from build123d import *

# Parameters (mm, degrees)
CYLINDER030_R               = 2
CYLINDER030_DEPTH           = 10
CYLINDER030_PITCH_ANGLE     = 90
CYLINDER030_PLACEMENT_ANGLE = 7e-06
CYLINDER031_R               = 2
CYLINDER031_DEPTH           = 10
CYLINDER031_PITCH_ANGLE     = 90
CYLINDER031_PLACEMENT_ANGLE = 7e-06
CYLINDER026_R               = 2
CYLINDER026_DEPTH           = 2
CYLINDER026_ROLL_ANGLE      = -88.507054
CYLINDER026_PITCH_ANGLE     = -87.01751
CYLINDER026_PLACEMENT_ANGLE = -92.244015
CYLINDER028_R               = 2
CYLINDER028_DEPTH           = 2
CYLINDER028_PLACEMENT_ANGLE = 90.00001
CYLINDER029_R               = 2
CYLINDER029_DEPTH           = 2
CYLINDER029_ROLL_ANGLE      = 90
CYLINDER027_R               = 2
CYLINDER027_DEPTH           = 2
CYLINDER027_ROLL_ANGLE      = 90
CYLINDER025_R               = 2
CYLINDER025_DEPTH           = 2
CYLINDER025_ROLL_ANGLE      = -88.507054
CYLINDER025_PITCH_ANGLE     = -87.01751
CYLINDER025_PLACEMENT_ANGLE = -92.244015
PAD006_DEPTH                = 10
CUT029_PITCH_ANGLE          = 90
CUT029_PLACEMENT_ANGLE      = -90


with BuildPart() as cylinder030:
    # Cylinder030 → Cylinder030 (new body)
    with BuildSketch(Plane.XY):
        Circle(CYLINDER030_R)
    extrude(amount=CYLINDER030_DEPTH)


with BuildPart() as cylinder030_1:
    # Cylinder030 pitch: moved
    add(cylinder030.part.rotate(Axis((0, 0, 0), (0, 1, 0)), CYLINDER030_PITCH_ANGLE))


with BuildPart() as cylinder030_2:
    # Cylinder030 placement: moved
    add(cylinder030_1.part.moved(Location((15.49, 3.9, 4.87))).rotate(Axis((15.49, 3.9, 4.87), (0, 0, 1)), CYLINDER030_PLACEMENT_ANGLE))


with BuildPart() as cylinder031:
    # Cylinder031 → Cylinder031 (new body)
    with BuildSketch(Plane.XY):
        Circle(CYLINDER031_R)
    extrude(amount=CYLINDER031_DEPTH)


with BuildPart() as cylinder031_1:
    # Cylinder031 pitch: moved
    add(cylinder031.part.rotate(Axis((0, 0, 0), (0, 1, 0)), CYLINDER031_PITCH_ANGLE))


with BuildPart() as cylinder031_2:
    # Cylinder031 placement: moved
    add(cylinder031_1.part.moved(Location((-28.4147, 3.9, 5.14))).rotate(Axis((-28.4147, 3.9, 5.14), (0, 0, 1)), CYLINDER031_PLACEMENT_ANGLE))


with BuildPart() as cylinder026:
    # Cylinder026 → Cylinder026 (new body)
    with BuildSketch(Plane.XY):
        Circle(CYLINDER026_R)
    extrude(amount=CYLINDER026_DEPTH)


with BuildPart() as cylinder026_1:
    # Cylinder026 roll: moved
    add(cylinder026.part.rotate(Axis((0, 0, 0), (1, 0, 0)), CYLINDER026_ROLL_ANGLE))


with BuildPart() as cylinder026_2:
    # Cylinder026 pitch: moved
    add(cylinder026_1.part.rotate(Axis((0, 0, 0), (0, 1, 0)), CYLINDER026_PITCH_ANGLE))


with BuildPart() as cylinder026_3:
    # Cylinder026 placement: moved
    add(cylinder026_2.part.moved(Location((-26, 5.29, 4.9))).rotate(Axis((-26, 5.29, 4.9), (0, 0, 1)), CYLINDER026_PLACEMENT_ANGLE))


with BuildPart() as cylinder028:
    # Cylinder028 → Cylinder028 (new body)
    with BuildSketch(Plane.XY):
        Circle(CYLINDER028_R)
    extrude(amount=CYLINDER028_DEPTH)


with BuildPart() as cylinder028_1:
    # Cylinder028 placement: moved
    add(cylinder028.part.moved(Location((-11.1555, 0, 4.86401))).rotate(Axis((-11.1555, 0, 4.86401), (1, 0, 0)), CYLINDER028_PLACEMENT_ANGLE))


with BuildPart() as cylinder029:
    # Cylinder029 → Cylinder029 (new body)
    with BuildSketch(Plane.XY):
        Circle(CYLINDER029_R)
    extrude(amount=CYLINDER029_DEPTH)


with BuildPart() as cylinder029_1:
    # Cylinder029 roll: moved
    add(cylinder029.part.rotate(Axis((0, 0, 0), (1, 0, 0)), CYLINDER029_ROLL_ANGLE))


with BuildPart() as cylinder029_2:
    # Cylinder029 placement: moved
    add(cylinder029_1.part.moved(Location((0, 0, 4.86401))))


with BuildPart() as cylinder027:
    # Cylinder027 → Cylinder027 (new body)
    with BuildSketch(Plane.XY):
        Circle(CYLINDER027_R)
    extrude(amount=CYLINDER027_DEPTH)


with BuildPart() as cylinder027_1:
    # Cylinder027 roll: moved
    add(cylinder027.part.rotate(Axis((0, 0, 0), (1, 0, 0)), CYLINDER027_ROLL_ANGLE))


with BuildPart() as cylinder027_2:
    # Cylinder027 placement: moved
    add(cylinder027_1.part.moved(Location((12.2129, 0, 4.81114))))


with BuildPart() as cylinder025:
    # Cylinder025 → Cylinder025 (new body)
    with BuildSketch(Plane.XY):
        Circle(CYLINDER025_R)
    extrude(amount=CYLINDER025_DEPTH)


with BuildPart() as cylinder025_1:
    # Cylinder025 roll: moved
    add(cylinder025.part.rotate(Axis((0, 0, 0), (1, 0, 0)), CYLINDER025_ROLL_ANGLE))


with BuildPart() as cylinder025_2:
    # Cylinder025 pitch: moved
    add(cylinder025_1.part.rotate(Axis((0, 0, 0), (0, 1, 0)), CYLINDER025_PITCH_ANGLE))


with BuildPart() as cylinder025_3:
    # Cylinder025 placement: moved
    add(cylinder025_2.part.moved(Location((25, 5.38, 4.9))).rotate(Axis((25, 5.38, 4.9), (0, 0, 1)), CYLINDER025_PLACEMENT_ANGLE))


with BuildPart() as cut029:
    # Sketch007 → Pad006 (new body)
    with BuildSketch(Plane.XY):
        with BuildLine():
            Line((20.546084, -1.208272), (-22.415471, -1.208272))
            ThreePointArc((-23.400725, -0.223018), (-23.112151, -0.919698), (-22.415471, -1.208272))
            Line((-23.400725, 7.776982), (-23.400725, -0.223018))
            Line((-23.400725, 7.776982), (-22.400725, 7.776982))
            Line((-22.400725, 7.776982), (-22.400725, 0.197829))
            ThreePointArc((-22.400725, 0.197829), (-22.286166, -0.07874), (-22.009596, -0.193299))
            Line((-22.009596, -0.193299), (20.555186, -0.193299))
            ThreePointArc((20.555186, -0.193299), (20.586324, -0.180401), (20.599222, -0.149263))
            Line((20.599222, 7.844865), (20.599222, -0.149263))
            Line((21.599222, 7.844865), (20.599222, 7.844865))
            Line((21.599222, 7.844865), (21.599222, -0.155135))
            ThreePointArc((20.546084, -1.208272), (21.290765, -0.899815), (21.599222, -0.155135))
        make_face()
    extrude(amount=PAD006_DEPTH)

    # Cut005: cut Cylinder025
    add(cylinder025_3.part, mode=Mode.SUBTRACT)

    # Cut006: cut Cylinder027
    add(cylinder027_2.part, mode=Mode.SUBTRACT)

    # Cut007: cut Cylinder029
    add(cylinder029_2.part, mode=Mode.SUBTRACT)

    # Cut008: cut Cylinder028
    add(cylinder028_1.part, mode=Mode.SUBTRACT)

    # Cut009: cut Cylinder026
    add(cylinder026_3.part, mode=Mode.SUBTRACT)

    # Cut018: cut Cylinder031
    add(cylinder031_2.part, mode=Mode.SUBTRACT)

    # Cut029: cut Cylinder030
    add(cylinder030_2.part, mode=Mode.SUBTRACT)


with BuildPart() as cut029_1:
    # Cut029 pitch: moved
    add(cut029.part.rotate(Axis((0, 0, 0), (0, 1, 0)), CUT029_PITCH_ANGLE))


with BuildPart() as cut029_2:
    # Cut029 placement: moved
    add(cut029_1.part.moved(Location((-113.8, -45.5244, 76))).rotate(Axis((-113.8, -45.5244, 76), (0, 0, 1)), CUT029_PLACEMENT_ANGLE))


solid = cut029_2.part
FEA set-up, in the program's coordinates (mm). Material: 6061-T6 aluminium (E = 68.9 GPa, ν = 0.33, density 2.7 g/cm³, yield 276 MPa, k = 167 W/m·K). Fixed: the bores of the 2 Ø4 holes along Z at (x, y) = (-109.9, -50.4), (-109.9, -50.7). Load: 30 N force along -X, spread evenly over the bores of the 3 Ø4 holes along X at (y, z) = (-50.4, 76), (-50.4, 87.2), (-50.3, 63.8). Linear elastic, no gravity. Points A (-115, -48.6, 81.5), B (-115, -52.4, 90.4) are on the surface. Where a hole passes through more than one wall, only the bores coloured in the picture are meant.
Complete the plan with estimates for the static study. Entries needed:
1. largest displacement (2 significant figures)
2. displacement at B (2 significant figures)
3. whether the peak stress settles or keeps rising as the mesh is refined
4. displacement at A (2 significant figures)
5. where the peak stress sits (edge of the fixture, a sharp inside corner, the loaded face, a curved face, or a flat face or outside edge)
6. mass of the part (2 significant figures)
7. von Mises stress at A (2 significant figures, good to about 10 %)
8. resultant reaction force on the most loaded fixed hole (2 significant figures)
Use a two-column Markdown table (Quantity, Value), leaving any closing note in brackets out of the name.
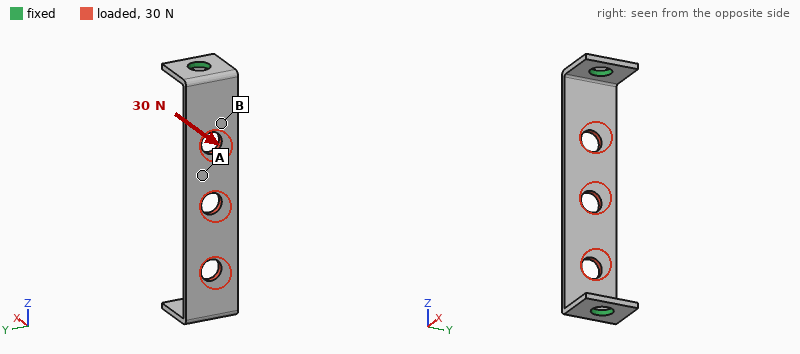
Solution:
| Quantity | Value |
|---|---|
| largest displacement | 0.18 mm |
| displacement at B | 0.070 mm |
| whether the peak stress settles or keeps rising as the mesh is refined | keeps rising |
| displacement at A | 0.16 mm |
| where the peak stress sits | a sharp inside corner |
| mass of the part | 1.5 g |
| von Mises stress at A | 32 MPa |
| resultant reaction force on the most loaded fixed hole | 50 N |
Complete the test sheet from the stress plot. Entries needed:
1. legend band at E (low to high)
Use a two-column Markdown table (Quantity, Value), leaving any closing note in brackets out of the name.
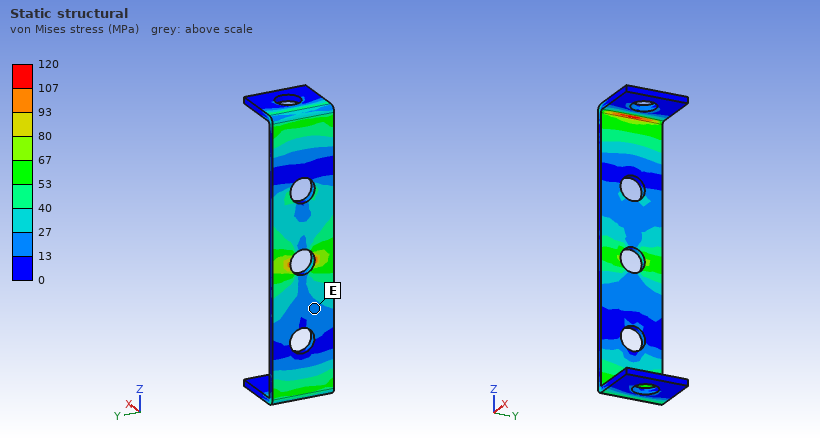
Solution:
| Quantity | Value |
|---|---|
| legend band at E | 13 to 27 MPa |
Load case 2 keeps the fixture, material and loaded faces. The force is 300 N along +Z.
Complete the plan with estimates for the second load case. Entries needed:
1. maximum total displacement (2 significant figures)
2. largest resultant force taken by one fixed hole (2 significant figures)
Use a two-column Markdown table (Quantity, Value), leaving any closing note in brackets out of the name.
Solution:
| Quantity | Value |
|---|---|
| maximum total displacement | 54 µm |
| largest resultant force taken by one fixed hole | 150 N |
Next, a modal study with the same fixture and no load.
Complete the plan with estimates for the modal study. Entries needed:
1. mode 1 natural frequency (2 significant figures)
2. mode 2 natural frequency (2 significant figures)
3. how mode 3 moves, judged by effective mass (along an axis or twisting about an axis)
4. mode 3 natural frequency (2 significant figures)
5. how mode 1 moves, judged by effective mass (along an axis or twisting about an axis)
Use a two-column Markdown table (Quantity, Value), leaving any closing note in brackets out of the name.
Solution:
| Quantity | Value |
|---|---|
| mode 1 natural frequency | 2600 Hz |
| mode 2 natural frequency | 6200 Hz |
| how mode 3 moves, judged by effective mass | twisting about Z |
| mode 3 natural frequency | 7200 Hz |
| how mode 1 moves, judged by effective mass | along X |
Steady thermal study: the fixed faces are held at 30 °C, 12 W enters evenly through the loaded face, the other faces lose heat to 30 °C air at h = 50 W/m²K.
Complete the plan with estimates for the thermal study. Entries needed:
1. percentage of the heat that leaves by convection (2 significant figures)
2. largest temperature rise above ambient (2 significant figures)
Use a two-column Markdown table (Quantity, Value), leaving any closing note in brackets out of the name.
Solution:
| Quantity | Value |
|---|---|
| percentage of the heat that leaves by convection | 15 % |
| largest temperature rise above ambient | 59 K |
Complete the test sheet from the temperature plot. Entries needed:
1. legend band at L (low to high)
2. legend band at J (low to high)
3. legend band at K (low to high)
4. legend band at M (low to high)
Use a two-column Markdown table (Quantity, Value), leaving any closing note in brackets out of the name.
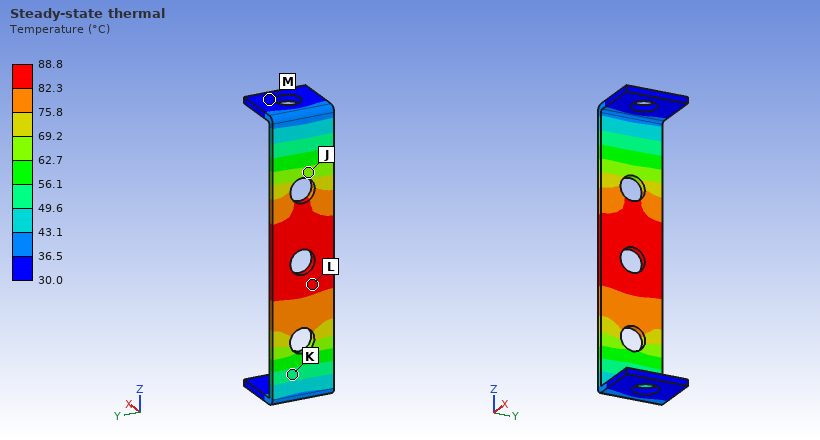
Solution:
| Quantity | Value |
|---|---|
| legend band at L | 82.3 to 88.8 °C |
| legend band at J | 62.7 to 69.2 °C |
| legend band at K | 49.6 to 56.1 °C |
| legend band at M | 30.0 to 36.5 °C |
